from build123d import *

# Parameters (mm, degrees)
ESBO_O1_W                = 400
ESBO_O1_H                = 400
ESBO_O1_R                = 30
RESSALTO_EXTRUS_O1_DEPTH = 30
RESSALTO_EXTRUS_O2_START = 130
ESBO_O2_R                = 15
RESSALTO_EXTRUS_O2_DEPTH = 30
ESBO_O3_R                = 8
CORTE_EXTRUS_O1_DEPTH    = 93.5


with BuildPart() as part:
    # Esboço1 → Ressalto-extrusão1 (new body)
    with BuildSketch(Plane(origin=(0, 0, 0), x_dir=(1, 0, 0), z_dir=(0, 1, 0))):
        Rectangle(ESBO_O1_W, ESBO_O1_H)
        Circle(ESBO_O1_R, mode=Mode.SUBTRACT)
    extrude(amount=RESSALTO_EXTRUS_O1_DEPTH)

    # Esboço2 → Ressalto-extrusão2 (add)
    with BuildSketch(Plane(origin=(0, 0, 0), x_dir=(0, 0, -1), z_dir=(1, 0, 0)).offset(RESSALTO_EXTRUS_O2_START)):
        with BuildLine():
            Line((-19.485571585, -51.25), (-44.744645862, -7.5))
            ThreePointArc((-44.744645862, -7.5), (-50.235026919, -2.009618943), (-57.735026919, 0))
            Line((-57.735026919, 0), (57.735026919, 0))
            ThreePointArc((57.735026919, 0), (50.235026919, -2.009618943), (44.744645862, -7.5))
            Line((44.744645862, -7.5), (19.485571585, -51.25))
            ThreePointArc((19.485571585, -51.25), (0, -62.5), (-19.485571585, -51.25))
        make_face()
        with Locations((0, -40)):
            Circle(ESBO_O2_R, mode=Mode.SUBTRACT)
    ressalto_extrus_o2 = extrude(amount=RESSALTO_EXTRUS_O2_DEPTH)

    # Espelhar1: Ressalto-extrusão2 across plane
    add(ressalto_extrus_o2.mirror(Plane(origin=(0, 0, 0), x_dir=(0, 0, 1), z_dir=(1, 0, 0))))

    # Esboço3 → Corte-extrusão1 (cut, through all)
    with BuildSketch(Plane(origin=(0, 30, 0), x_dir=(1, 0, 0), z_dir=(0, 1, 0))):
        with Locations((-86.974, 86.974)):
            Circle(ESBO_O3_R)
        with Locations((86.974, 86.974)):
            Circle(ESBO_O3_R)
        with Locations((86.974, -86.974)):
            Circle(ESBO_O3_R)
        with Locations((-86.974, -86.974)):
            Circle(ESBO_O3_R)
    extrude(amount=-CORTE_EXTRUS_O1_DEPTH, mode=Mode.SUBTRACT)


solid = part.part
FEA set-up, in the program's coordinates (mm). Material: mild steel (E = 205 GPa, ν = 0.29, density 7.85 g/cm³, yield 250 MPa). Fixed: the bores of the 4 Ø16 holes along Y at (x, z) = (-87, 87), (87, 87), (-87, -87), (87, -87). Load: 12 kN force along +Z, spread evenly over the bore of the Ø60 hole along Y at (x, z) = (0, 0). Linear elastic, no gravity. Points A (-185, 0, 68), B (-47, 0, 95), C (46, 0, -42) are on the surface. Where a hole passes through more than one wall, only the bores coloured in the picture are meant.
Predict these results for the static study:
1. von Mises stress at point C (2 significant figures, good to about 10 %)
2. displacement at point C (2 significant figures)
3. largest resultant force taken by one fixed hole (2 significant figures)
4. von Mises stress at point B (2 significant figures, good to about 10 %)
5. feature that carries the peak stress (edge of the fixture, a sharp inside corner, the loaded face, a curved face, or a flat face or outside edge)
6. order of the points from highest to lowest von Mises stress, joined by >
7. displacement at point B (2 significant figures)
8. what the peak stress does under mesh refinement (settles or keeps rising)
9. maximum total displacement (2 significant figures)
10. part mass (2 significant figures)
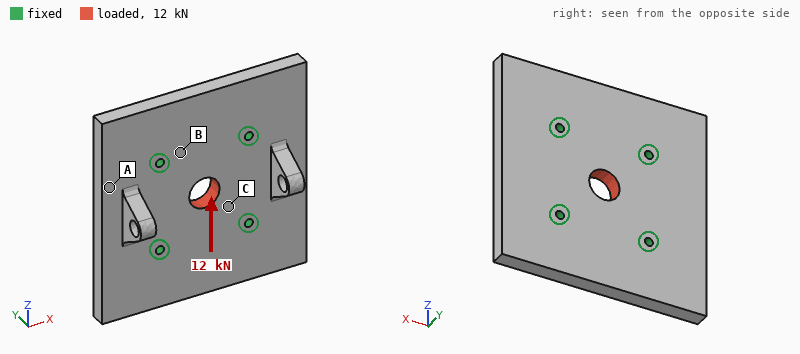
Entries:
1.5 MPa
0.52 µm
3.1 kN
0.86 MPa
edge of the fixture
C > B > A
0.39 µm
keeps rising
0.99 µm
38 kg
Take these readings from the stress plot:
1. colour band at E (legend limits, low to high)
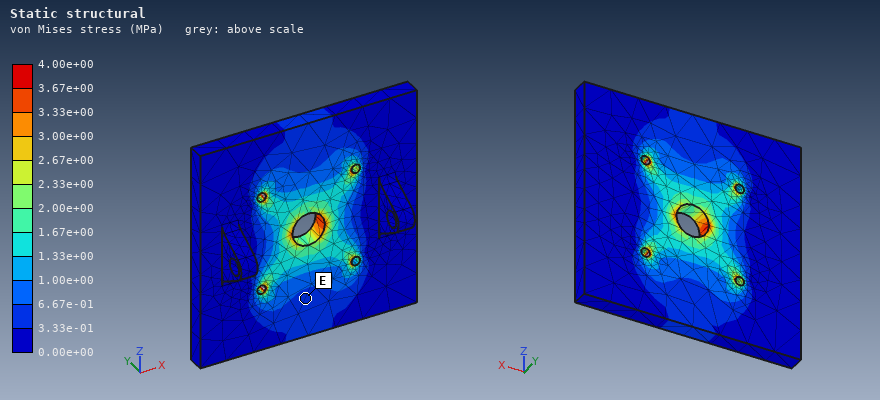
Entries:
3.33e-01 to 6.67e-01 MPa
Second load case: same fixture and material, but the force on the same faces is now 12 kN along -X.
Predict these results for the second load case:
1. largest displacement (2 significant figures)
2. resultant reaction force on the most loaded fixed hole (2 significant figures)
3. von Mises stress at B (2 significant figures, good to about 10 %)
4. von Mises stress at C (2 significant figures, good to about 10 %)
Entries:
0.99 µm
3.1 kN
0.58 MPa
1.5 MPa
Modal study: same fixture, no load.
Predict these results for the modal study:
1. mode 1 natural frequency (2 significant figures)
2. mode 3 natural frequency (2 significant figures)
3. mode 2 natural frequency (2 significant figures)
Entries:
1300 Hz
1400 Hz
1300 Hz
